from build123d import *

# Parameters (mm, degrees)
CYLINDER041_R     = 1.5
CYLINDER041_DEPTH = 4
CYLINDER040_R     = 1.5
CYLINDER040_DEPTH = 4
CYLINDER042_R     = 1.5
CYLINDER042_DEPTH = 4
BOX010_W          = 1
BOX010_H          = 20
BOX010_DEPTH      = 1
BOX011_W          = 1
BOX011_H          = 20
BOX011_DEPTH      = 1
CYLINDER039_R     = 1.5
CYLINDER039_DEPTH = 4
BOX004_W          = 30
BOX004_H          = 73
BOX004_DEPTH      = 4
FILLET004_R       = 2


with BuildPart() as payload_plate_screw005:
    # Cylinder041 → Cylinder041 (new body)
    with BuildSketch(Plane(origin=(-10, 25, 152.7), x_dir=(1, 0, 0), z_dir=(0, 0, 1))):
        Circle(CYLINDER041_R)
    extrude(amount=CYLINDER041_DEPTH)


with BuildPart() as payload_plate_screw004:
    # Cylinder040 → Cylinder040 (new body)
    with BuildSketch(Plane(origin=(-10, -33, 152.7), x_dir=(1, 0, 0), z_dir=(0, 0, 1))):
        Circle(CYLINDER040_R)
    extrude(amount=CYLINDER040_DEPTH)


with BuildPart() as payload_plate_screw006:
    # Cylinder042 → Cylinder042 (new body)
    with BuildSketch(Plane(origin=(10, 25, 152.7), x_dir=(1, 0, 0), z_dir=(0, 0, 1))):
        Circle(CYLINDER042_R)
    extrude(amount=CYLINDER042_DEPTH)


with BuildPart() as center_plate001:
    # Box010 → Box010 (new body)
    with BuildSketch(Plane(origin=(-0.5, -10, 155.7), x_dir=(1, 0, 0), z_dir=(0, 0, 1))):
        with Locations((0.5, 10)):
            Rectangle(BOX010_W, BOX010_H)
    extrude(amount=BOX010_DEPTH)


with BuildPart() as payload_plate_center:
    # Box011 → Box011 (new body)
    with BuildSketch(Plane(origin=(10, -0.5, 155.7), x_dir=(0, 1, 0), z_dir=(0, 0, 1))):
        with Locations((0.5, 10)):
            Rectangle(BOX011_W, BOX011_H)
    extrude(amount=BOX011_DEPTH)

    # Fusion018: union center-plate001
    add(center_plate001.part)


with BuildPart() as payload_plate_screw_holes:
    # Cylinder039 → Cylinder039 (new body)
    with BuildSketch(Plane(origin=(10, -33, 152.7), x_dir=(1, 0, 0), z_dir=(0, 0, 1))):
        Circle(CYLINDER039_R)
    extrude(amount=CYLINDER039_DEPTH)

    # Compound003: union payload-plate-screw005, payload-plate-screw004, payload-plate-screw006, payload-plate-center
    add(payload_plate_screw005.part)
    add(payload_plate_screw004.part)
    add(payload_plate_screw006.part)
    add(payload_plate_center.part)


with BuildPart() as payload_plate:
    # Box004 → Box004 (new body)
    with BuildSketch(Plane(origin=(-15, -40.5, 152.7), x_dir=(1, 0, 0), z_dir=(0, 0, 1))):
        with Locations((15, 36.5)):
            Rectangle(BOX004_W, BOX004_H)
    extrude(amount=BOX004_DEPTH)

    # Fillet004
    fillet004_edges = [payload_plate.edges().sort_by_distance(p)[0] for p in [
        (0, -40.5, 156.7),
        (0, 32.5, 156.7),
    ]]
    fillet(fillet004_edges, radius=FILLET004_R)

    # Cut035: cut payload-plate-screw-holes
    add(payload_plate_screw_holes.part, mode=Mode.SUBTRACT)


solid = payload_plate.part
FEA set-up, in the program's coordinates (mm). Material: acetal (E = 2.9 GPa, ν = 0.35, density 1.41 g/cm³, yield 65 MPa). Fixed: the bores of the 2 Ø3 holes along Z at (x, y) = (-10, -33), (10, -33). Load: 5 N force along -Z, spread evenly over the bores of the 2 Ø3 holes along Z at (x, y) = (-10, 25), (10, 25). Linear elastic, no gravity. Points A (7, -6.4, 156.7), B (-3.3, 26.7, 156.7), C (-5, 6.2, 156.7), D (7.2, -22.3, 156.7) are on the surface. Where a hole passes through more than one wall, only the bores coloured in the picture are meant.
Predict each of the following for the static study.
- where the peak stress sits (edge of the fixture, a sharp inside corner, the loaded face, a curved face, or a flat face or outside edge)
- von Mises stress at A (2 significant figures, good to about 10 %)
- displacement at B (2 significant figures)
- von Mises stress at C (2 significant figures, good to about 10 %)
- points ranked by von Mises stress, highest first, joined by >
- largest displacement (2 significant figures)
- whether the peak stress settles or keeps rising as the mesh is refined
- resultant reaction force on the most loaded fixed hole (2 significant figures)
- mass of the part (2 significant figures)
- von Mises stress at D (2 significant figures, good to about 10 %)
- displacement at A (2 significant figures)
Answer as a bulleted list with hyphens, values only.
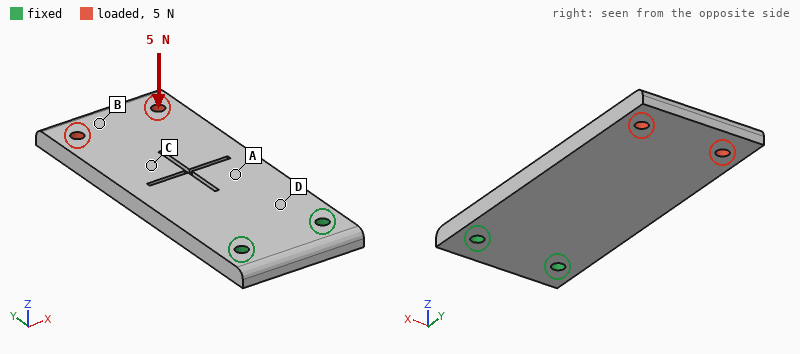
- edge of the fixture
- 1.9 MPa
- 0.76 mm
- 1.1 MPa
- D > A > C > B
- 0.86 mm
- keeps rising
- 2.5 N
- 12 g
- 2.8 MPa
- 0.20 mm
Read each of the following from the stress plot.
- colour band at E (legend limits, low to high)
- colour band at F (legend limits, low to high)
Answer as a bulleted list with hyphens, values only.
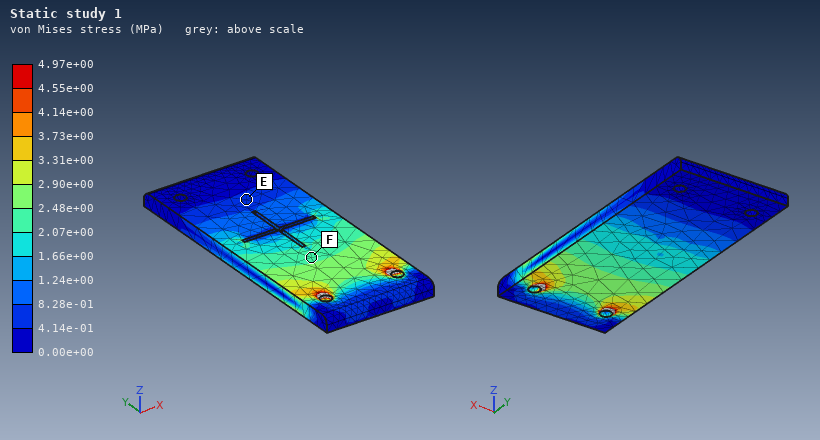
- 4.14e-01 to 8.28e-01 MPa
- 2.07e+00 to 2.48e+00 MPa
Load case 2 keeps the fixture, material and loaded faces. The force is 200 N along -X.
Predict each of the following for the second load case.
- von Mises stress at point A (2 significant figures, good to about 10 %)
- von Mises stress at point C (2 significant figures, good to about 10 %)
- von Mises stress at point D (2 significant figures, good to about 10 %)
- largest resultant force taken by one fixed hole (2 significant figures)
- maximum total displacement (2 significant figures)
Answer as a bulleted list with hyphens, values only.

- 5.7 MPa
- 4.4 MPa
- 8.8 MPa
- 560 N
- 0.77 mm
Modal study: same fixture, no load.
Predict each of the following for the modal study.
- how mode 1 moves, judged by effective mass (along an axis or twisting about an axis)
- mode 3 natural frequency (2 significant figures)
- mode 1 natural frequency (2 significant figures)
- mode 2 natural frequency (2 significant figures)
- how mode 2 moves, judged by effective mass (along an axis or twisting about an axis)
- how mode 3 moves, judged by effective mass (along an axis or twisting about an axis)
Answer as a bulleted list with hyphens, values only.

- along Z
- 1300 Hz
- 220 Hz
- 950 Hz
- twisting about Y
- along Z
